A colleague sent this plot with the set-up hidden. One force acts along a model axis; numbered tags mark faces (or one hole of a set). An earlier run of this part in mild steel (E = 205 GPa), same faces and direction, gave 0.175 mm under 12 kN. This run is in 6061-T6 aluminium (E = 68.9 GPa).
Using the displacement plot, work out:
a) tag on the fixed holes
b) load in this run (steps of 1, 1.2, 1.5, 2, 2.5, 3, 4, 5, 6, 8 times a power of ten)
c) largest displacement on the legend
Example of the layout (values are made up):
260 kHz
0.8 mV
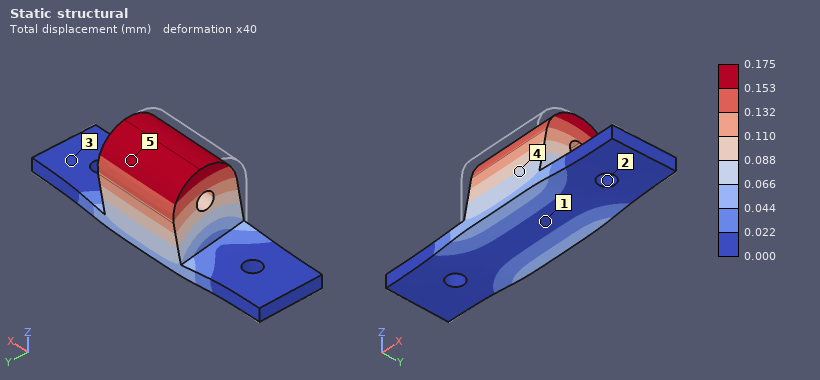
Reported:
2
4 kN
0.175 mm
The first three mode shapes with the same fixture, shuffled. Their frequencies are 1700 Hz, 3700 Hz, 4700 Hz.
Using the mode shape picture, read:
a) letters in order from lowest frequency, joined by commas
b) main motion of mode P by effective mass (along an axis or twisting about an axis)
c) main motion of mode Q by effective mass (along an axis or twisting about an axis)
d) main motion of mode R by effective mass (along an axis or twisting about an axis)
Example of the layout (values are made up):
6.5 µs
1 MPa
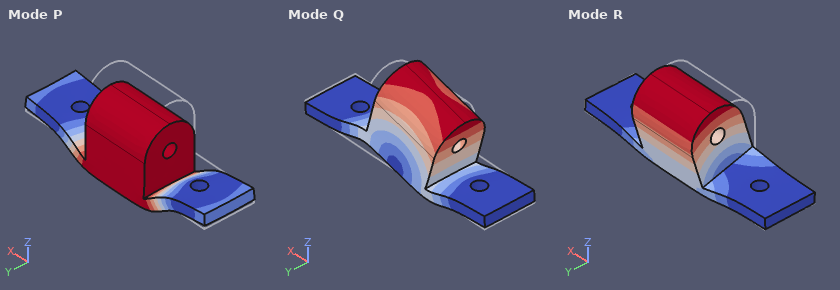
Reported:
R, P, Q
along Z
along X
along Y
